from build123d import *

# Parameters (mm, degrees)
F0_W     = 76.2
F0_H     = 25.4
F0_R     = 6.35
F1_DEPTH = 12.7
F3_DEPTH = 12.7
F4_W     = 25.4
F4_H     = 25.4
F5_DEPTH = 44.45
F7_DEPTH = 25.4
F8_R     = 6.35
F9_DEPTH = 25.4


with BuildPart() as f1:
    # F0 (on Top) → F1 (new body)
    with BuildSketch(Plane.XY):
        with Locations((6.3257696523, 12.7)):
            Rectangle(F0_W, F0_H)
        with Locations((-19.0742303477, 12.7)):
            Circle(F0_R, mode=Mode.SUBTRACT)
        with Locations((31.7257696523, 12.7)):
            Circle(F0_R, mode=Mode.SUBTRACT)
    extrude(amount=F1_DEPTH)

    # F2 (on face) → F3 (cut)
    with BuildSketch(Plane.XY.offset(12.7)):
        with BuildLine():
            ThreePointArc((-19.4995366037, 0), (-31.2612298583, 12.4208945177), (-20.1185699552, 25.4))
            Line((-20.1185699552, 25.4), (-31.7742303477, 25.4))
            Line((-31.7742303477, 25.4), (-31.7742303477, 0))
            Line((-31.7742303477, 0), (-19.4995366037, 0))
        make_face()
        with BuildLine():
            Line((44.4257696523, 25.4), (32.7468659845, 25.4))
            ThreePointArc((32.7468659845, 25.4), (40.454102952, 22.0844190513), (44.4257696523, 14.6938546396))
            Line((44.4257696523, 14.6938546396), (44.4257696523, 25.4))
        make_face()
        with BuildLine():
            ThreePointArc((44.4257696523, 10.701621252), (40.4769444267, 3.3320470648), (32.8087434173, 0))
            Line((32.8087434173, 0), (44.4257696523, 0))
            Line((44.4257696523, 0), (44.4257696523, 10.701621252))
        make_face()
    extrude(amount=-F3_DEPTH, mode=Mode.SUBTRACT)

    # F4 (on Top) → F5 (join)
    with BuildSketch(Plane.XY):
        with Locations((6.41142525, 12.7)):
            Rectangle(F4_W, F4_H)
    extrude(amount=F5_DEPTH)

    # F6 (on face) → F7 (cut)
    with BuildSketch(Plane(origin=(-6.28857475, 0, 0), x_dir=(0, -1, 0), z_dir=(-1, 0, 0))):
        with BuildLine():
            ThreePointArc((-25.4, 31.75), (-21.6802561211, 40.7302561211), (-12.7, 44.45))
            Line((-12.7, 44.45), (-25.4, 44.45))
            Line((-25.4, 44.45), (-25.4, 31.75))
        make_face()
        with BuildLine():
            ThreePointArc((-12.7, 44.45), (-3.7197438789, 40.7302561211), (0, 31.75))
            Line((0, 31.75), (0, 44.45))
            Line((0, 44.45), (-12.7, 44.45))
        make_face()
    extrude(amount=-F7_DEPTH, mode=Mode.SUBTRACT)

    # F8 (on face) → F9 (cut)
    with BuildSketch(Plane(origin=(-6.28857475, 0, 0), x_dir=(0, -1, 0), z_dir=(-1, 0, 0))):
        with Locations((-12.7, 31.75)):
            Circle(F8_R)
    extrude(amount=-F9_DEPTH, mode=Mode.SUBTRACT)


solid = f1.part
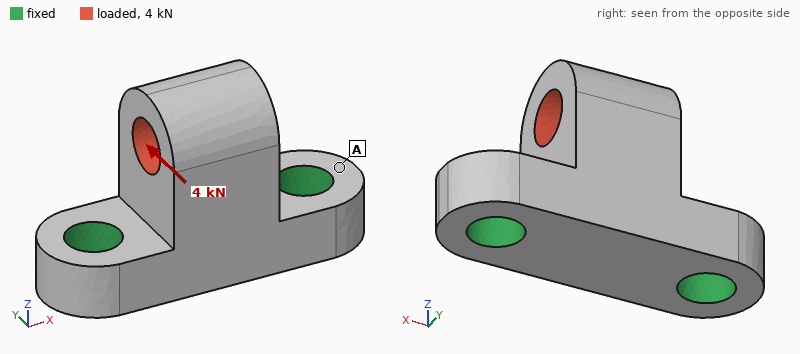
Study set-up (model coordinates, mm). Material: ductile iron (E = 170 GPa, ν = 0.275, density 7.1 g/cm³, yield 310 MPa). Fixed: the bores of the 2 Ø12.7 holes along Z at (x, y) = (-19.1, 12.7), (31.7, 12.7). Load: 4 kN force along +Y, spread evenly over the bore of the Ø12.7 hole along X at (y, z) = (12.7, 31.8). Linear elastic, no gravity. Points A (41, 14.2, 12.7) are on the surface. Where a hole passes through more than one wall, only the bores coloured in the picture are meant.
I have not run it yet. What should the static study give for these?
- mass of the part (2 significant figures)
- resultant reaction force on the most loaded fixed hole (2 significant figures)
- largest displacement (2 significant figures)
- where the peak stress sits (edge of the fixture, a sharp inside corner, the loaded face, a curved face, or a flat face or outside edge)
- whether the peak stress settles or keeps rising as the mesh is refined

250 g
2.0 kN
35 µm
edge of the fixture
keeps rising
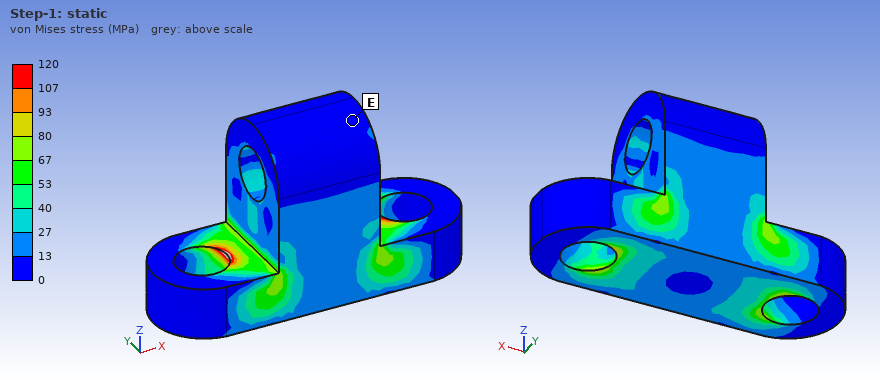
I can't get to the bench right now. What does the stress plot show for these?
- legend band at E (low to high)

0 to 13 MPa
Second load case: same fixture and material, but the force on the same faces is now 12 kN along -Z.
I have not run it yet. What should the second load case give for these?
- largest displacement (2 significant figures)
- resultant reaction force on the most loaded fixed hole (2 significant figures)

11 µm
6.3 kN
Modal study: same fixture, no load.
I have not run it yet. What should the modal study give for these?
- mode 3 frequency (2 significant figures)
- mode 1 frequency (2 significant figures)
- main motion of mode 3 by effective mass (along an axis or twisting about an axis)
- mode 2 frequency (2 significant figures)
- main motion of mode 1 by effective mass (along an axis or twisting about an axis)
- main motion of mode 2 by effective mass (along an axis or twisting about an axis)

16 kHz
6800 Hz
along Z
12 kHz
along Y
along X
